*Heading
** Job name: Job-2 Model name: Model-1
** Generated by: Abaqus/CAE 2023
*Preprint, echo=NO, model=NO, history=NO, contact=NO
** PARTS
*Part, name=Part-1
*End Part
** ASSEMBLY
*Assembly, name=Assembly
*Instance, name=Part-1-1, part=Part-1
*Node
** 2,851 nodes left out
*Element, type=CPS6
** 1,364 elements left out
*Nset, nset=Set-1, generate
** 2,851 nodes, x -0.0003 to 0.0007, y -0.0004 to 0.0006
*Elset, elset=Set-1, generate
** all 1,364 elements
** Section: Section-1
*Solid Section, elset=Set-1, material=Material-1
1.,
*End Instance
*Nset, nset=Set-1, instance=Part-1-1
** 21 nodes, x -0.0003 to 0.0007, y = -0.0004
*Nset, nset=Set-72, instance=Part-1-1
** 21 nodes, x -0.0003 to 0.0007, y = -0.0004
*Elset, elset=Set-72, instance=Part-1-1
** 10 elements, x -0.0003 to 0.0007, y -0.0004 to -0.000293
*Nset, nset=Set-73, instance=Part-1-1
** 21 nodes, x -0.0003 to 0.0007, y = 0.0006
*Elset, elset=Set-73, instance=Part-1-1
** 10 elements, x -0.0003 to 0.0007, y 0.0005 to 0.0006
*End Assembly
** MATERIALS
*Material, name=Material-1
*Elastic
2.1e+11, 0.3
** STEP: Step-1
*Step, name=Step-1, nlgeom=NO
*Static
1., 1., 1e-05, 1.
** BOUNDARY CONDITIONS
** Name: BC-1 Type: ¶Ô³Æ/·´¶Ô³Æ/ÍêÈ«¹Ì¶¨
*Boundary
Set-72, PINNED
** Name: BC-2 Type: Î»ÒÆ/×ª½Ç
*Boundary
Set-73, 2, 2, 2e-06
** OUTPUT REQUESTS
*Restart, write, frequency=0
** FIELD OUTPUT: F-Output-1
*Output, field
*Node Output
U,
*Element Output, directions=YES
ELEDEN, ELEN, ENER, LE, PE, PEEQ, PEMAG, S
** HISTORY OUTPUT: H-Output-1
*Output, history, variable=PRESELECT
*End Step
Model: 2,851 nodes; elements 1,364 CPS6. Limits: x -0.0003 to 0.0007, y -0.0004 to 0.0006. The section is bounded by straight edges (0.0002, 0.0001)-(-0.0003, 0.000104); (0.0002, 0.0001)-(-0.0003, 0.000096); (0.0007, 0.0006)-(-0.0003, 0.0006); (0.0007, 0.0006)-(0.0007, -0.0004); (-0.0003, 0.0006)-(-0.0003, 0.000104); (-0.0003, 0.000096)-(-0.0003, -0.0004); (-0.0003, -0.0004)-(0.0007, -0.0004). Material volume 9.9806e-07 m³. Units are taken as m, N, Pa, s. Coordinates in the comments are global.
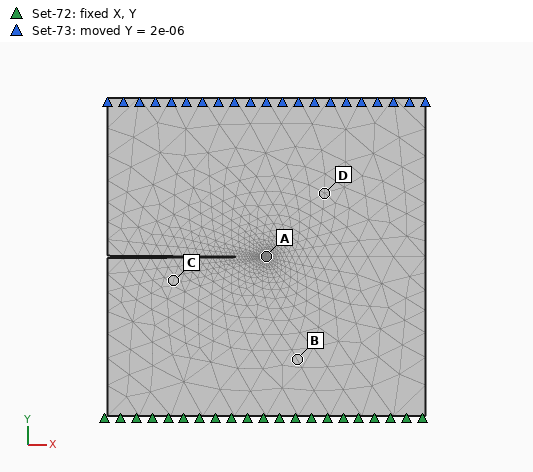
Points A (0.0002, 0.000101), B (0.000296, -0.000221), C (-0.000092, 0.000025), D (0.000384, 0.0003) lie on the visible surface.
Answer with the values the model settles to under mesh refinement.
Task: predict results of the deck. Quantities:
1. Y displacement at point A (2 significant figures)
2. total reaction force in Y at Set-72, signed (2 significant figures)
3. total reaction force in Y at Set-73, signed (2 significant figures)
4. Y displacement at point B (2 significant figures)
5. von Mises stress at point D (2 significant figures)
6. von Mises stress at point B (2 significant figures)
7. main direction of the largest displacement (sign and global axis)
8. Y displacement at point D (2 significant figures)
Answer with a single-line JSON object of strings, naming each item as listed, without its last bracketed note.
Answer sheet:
{"Y displacement at point A": "1.0e-06 m", "total reaction force in Y at Set-72, signed": "-2.6e+05 N", "total reaction force in Y at Set-73, signed": "2.6e+05 N", "Y displacement at point B": "2.9e-07 m", "von Mises stress at point D": "4.5e+08 Pa", "von Mises stress at point B": "3.7e+08 Pa", "main direction of the largest displacement": "+Y", "Y displacement at point D": "1.4e-06 m"}
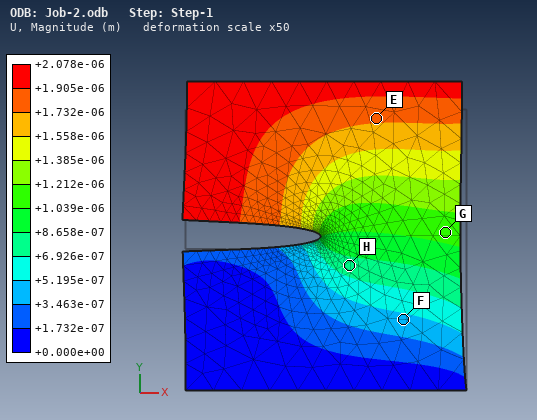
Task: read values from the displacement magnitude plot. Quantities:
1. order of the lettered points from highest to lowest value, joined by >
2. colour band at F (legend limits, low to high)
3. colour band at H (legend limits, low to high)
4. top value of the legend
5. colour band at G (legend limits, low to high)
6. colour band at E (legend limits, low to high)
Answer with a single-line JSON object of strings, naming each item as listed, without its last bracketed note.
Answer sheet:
{"order of the lettered points from highest to lowest value, joined by >": "E > G > H > F", "colour band at F": "+3.463e-07 to +5.195e-07 m", "colour band at H": "+6.926e-07 to +8.658e-07 m", "top value of the legend": "+2.078e-06 m", "colour band at G": "+1.039e-06 to +1.212e-06 m", "colour band at E": "+1.732e-06 to +1.905e-06 m"}
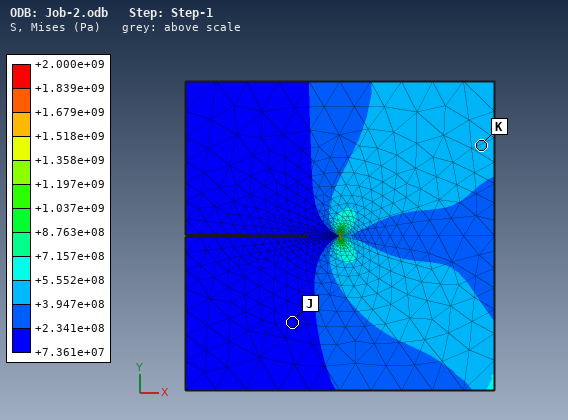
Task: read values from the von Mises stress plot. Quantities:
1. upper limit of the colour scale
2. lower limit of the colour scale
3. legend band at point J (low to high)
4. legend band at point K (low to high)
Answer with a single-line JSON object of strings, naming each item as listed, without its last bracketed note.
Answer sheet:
{"upper limit of the colour scale": "+2.000e+09 Pa", "lower limit of the colour scale": "+7.361e+07 Pa", "legend band at point J": "+7.361e+07 to +2.341e+08 Pa", "legend band at point K": "+3.947e+08 to +5.552e+08 Pa"}
